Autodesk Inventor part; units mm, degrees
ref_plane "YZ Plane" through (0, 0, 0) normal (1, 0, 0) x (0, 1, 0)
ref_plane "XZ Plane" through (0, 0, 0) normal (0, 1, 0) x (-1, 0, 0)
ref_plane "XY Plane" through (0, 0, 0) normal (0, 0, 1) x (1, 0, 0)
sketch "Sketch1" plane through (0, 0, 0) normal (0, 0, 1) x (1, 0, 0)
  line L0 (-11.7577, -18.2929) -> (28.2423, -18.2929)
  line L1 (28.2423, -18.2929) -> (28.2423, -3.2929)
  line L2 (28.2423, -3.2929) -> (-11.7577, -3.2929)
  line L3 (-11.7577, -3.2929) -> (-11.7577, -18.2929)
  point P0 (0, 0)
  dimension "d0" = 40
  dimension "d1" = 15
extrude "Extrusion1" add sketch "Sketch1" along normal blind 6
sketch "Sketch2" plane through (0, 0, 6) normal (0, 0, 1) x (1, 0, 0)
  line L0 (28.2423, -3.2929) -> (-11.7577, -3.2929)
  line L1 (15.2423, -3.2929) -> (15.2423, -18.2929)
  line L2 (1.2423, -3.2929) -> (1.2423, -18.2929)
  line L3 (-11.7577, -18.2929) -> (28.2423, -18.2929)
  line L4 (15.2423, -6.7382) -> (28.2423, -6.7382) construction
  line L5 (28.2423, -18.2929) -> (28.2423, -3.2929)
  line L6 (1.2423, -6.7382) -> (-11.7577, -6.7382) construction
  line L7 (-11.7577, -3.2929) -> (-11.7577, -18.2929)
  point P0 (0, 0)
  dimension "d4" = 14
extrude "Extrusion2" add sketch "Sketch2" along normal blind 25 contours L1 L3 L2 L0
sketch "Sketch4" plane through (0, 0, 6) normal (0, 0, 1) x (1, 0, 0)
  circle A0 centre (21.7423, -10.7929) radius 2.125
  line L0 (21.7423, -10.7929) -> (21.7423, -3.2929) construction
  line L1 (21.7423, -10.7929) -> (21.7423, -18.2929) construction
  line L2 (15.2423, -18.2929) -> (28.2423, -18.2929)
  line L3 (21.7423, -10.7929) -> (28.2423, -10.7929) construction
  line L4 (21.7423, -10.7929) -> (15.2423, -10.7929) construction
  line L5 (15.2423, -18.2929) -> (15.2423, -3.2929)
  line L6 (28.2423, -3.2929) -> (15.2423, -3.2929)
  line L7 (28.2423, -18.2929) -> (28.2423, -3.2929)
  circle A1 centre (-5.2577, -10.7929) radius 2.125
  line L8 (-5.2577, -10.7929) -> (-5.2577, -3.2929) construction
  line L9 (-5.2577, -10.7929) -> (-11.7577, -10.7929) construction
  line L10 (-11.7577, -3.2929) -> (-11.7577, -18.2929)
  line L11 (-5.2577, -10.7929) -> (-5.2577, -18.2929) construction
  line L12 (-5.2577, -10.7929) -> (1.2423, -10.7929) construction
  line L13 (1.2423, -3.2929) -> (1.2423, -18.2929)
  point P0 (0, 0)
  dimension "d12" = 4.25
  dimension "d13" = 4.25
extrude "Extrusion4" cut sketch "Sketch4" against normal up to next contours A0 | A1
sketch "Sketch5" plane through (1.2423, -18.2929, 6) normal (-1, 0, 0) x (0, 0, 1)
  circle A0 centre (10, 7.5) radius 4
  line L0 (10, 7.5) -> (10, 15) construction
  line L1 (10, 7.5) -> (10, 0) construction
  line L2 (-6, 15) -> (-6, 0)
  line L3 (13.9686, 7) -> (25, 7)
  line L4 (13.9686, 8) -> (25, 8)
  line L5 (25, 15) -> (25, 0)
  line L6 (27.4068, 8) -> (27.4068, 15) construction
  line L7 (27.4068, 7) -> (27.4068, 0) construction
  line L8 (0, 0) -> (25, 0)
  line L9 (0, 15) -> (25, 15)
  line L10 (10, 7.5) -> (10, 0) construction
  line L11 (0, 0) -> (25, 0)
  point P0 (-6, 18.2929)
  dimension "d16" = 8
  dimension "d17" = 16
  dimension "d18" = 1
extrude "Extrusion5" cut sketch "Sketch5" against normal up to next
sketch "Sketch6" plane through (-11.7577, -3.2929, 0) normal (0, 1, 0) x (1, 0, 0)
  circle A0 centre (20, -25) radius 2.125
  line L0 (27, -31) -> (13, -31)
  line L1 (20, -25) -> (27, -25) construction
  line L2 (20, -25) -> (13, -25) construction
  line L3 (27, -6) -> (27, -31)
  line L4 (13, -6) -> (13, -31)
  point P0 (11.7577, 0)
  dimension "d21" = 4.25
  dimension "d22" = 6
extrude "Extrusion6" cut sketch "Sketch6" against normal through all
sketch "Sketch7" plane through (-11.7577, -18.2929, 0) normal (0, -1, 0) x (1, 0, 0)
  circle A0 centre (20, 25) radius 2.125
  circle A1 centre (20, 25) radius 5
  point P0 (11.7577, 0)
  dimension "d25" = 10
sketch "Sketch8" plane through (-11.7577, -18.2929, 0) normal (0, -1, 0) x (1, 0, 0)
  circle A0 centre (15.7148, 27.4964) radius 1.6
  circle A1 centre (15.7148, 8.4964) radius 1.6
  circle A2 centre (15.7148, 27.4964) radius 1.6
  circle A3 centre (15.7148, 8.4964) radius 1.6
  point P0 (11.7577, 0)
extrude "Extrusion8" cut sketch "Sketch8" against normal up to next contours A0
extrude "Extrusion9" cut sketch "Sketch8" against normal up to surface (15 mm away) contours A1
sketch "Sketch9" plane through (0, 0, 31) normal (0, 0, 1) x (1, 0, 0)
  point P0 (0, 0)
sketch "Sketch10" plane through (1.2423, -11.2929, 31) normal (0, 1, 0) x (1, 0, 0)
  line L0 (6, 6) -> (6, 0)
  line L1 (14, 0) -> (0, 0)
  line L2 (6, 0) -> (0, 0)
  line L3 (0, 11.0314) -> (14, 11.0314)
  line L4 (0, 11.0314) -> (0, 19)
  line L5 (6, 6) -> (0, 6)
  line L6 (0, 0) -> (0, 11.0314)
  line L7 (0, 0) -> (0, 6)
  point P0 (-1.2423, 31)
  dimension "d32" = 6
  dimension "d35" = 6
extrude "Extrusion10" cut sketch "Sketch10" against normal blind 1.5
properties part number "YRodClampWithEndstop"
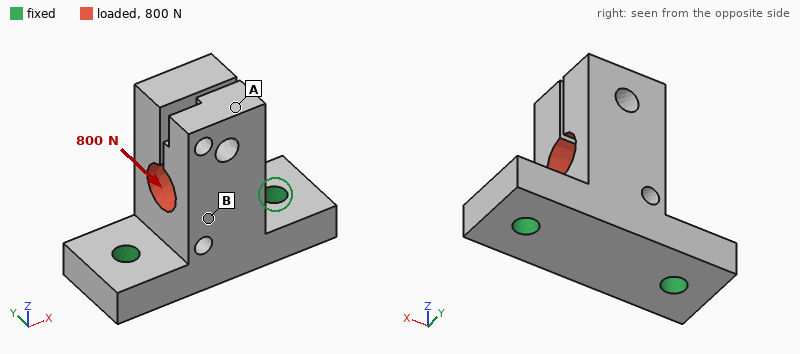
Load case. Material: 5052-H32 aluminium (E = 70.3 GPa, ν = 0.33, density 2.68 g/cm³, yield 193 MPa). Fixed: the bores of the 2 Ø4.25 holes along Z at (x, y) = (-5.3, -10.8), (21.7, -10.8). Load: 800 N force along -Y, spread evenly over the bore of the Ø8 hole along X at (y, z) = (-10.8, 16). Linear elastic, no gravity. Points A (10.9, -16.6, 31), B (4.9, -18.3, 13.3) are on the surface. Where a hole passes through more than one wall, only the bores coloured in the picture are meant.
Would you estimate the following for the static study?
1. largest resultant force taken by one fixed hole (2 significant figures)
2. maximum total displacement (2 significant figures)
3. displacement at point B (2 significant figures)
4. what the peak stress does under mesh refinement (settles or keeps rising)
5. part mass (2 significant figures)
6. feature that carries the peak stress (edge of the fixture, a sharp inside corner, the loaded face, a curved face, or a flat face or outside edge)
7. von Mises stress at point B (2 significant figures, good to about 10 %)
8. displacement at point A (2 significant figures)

400 N
75 µm
26 µm
keeps rising
20 g
edge of the fixture
18 MPa
73 µm
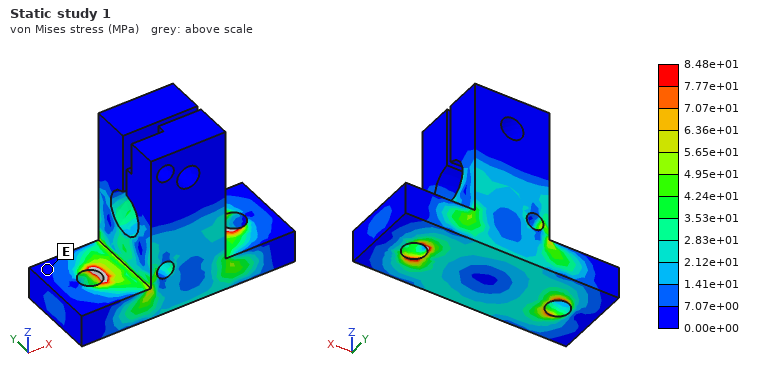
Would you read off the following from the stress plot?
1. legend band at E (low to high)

0.00e+00 to 7.07e+00 MPa
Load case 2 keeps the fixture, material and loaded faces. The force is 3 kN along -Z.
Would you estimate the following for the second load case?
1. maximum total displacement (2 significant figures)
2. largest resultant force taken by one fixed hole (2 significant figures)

69 µm
1.6 kN
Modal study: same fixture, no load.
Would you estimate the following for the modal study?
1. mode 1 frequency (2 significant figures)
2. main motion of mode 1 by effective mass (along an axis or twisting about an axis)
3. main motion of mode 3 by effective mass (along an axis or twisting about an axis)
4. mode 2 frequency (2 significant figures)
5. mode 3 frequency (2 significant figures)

4700 Hz
along Y
along X
6300 Hz
9700 Hz
